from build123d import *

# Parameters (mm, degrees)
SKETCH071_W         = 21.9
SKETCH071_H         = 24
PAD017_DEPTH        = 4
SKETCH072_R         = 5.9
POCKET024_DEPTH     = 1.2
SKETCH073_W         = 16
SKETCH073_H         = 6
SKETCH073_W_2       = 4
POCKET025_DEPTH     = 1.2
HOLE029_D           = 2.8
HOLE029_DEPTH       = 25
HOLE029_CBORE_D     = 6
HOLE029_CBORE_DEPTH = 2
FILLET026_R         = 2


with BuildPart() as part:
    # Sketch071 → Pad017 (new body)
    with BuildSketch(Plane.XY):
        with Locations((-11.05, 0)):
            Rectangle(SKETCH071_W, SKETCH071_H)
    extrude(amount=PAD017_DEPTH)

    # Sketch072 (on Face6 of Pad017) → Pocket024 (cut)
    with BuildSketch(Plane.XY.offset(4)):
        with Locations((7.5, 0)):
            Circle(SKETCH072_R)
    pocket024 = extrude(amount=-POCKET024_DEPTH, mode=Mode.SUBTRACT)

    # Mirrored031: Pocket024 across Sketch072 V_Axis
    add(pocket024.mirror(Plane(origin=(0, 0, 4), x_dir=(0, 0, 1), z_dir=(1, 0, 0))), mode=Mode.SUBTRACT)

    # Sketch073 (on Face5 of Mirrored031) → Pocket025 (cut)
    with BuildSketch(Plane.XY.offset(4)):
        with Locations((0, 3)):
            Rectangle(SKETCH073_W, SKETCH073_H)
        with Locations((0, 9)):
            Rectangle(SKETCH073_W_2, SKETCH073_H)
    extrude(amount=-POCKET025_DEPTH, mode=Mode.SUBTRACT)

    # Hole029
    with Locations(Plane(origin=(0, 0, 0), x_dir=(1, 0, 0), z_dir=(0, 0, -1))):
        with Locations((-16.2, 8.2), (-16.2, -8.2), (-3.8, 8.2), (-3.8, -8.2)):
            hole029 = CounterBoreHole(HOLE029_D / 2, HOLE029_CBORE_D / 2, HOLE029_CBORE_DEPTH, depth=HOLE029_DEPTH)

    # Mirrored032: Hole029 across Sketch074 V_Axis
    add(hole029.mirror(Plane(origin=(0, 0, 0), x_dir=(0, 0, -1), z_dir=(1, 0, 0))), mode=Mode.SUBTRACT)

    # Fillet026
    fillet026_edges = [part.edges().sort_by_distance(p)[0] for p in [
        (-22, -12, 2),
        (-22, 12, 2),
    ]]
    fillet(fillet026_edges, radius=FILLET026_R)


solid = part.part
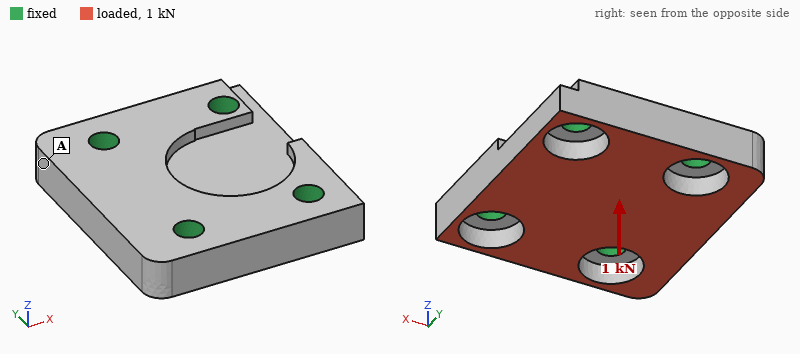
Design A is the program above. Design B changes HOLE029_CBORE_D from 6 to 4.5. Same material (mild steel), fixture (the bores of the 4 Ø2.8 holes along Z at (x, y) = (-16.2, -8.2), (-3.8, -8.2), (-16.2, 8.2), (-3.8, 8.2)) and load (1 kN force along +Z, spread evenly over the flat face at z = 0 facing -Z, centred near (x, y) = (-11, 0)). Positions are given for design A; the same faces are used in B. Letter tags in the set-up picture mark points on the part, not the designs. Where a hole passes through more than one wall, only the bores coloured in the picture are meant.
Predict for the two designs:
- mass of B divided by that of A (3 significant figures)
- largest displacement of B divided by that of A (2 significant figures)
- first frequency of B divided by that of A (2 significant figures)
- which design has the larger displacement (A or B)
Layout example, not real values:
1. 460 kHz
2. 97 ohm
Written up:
1. 1.06
2. 0.82
3. 1.1
4. A
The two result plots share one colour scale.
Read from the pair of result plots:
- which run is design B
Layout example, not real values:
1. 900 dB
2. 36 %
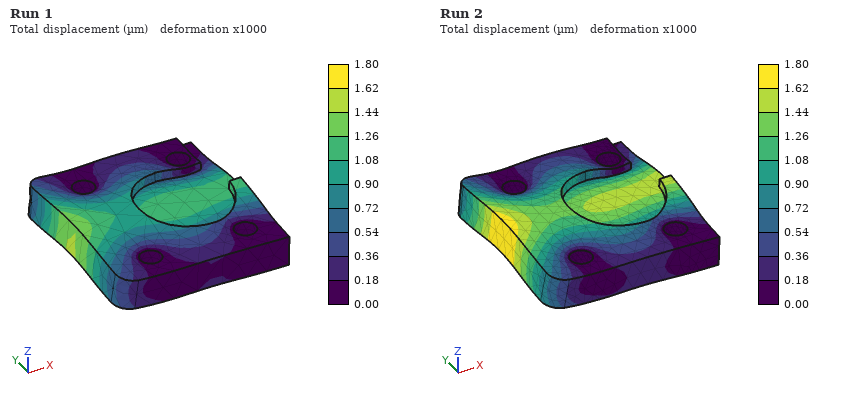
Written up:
1. Run 1
